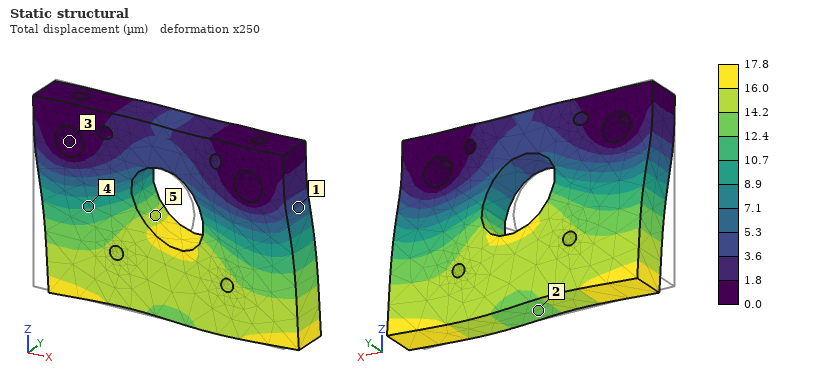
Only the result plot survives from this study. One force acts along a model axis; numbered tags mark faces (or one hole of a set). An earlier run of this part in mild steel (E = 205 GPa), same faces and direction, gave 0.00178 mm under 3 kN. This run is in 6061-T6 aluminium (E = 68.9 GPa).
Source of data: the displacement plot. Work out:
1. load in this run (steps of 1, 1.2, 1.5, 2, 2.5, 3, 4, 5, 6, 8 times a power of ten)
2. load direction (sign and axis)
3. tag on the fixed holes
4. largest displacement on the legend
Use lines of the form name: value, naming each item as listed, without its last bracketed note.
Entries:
load in this run: 10 kN
load direction: +X
tag on the fixed holes: 3
largest displacement on the legend: 17.8 µm
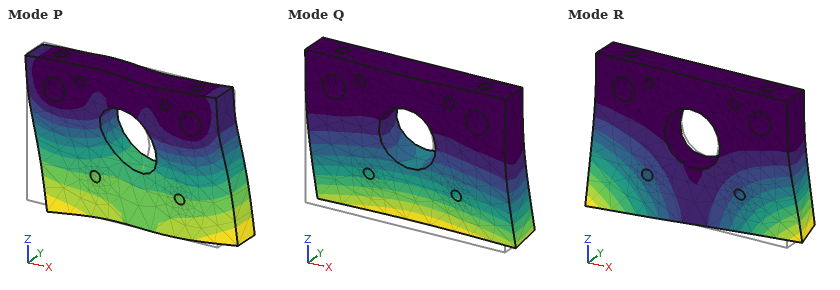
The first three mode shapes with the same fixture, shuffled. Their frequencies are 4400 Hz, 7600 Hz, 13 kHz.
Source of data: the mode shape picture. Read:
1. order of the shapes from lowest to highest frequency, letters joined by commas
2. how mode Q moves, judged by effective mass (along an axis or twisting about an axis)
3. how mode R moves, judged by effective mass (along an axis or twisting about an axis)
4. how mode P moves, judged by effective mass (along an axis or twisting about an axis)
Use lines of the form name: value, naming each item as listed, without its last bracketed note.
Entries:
order of the shapes from lowest to highest frequency, letters joined by commas: Q, R, P
how mode Q moves, judged by effective mass: along Y
how mode R moves, judged by effective mass: twisting about Z
how mode P moves, judged by effective mass: along X
